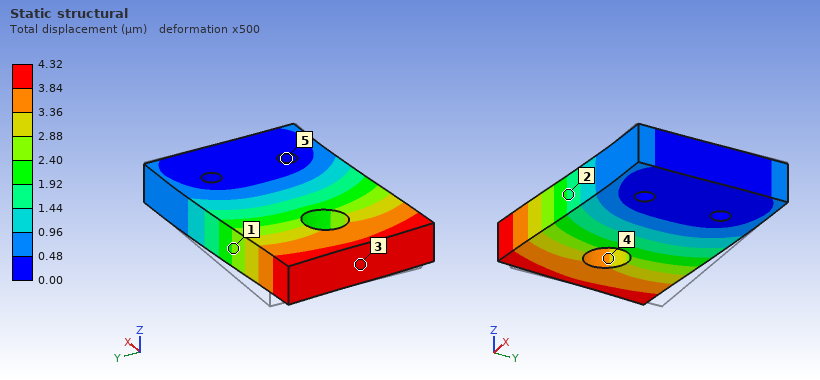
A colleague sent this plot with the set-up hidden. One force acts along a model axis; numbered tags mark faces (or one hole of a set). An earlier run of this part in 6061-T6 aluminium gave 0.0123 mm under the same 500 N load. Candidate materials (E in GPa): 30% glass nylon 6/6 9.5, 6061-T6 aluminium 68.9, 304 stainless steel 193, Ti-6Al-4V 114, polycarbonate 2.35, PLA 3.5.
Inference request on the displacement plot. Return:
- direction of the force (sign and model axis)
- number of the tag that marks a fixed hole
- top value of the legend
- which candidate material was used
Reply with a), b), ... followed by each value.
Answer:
a) -Y
b) 5
c) 4.32 µm
d) 304 stainless steel
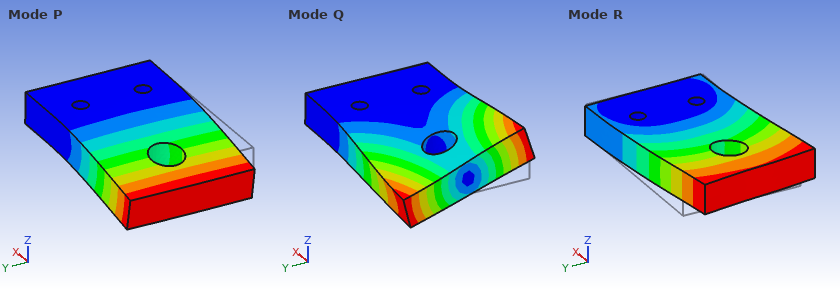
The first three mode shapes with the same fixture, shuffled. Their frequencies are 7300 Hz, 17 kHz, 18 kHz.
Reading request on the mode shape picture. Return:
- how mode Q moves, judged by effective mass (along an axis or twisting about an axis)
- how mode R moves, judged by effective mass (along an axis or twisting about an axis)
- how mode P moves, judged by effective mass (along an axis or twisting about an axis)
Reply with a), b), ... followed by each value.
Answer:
a) twisting about X
b) along Y
c) along Z
